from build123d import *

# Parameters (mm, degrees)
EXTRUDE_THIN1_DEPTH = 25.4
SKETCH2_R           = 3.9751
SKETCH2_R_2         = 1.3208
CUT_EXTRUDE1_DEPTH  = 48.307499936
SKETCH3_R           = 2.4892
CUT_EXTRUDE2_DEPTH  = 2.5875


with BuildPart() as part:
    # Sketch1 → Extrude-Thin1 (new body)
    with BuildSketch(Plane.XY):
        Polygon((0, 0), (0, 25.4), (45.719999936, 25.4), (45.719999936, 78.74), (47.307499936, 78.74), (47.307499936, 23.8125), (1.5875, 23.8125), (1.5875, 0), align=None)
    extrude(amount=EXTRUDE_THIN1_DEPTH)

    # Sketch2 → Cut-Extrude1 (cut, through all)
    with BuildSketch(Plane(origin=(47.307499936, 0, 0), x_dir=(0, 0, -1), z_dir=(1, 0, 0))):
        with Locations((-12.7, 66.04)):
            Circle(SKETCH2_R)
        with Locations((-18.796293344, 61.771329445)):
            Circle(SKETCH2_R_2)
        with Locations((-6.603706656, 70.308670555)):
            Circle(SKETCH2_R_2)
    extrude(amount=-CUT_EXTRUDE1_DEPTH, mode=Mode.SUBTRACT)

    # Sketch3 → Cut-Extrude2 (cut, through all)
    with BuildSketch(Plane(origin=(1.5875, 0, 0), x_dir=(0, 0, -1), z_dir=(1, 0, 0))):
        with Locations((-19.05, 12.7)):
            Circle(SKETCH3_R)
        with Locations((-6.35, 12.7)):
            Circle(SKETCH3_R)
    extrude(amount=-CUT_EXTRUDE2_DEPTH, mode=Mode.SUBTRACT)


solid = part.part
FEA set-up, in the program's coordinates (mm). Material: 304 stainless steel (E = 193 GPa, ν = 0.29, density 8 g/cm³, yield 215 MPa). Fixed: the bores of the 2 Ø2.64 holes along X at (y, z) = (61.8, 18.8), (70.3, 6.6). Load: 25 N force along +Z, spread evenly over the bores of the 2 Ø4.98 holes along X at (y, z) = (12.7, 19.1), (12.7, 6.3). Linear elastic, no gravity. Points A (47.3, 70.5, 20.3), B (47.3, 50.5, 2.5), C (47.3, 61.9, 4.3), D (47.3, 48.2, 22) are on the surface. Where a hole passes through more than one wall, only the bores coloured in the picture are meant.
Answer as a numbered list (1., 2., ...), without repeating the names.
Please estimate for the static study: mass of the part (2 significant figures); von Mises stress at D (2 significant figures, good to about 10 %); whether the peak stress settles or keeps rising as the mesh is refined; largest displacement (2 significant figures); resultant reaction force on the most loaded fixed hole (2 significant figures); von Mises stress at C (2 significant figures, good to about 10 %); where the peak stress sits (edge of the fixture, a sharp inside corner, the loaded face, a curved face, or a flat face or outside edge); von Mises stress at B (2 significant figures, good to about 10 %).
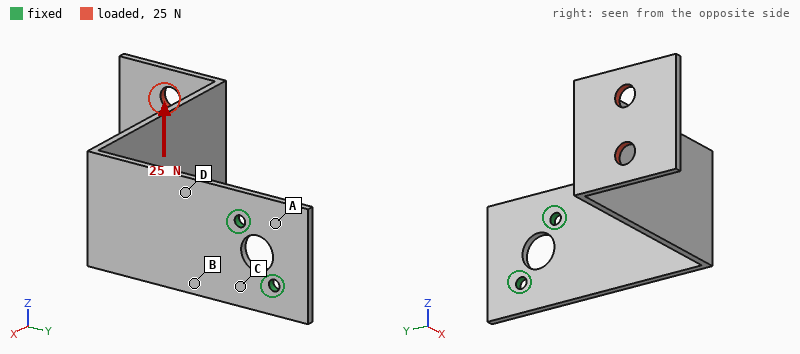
1. 39 g
2. 96 MPa
3. keeps rising
4. 0.87 mm
5. 93 N
6. 66 MPa
7. edge of the fixture
8. 81 MPa
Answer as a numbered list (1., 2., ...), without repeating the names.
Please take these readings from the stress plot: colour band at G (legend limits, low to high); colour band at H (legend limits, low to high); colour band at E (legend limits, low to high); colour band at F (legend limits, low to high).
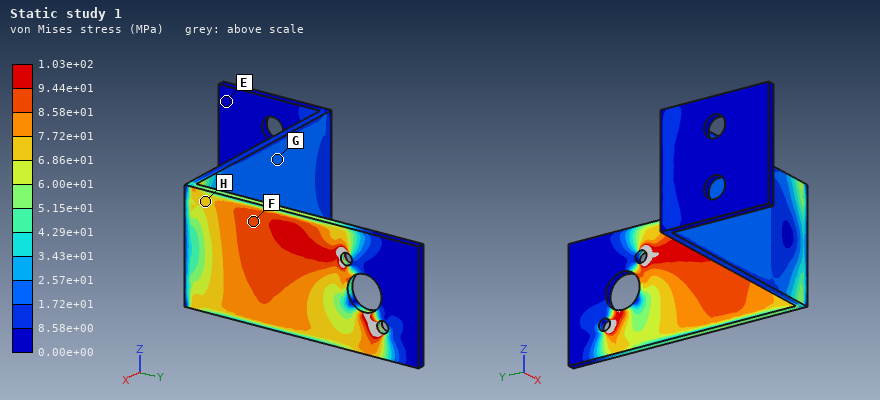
1. 1.72e+01 to 2.57e+01 MPa
2. 6.86e+01 to 7.72e+01 MPa
3. 0.00e+00 to 8.58e+00 MPa
4. 8.58e+01 to 9.44e+01 MPa
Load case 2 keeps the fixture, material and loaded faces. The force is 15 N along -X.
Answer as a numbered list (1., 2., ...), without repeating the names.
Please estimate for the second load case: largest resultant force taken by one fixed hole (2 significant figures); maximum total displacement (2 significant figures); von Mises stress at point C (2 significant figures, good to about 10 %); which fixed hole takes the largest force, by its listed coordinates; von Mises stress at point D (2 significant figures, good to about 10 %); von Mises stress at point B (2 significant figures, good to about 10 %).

1. 28 N
2. 0.92 mm
3. 42 MPa
4. (61.8, 18.8)
5. 52 MPa
6. 48 MPa
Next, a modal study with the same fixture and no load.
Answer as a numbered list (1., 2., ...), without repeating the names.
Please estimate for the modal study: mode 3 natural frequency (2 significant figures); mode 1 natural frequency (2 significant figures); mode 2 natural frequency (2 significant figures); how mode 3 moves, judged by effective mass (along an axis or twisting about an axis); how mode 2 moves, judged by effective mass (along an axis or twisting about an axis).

1. 520 Hz
2. 150 Hz
3. 260 Hz
4. along X
5. along Z
